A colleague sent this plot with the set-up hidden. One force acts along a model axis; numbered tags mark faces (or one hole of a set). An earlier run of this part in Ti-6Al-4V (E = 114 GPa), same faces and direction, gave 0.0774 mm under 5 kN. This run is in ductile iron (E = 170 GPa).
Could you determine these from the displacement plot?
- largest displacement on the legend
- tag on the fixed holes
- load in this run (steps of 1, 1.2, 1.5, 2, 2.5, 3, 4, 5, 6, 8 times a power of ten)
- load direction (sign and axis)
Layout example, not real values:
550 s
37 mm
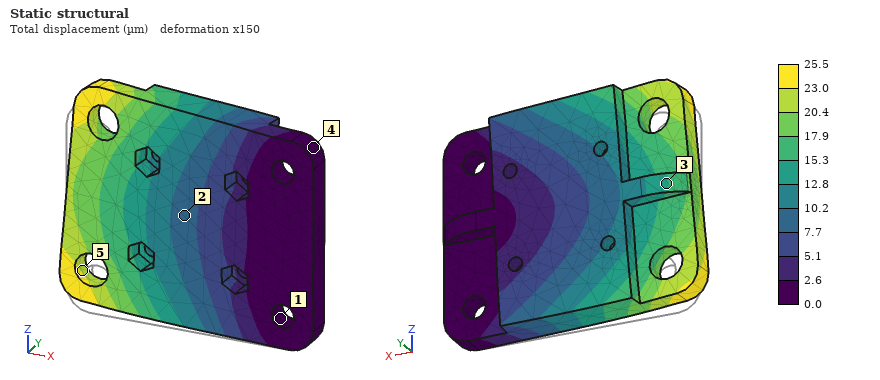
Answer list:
25.5 µm
1
2.5 kN
+Z
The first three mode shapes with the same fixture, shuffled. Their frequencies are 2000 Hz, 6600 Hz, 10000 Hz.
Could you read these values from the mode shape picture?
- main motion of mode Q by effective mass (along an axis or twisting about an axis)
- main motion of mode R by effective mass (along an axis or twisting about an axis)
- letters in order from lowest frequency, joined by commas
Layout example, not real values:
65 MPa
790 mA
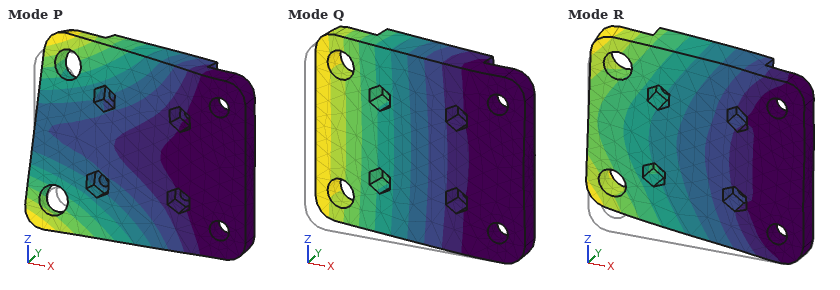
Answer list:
along Y
along Z
Q, P, R
